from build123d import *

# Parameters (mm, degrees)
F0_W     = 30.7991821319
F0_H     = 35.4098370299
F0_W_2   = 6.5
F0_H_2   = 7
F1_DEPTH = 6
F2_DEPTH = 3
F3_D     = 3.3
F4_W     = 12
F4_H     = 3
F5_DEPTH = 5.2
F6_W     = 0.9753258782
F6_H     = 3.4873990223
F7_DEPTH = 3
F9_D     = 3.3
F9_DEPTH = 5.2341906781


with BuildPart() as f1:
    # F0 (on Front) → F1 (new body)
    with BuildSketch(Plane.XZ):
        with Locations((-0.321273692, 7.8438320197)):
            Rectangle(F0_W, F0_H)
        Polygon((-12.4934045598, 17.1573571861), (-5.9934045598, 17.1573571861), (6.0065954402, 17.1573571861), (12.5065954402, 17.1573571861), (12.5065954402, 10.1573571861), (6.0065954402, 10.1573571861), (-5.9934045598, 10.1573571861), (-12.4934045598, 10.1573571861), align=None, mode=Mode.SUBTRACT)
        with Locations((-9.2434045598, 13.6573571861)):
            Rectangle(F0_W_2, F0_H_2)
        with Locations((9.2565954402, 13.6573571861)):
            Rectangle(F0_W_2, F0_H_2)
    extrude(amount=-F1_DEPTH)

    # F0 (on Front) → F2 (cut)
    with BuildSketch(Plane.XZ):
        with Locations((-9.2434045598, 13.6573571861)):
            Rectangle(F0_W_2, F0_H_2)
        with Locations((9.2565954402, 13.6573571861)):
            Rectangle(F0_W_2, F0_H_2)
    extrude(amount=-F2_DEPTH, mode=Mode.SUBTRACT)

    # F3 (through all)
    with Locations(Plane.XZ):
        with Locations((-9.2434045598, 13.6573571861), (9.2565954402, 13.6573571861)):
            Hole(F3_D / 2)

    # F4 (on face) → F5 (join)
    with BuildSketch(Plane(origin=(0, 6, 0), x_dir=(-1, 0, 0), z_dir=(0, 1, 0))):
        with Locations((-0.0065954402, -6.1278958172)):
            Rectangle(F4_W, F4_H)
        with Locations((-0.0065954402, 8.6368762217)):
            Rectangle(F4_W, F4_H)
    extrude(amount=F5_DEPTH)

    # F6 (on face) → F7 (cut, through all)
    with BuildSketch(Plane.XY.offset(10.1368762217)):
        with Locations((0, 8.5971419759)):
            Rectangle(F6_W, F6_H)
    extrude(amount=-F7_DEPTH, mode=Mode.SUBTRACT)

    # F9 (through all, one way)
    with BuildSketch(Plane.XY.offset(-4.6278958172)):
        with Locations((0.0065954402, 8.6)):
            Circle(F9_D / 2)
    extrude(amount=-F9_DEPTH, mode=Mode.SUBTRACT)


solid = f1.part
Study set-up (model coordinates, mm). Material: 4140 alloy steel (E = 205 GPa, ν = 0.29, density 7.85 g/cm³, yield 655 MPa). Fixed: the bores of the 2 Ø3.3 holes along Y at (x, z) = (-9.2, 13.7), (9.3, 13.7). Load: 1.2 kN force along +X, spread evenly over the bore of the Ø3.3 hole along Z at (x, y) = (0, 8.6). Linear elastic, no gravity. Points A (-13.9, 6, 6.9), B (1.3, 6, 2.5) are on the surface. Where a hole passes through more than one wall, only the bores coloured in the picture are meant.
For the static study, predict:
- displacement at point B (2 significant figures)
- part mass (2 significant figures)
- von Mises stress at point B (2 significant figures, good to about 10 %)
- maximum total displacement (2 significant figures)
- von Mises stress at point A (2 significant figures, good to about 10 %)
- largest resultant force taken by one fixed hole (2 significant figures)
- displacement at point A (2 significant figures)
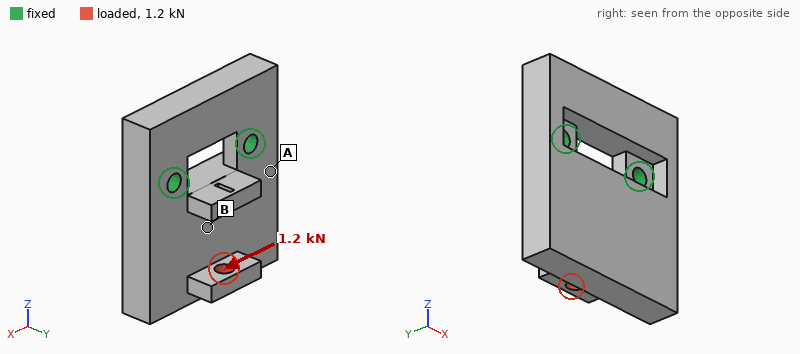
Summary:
4.8 µm
48 g
59 MPa
18 µm
22 MPa
1.2 kN
4.9 µm
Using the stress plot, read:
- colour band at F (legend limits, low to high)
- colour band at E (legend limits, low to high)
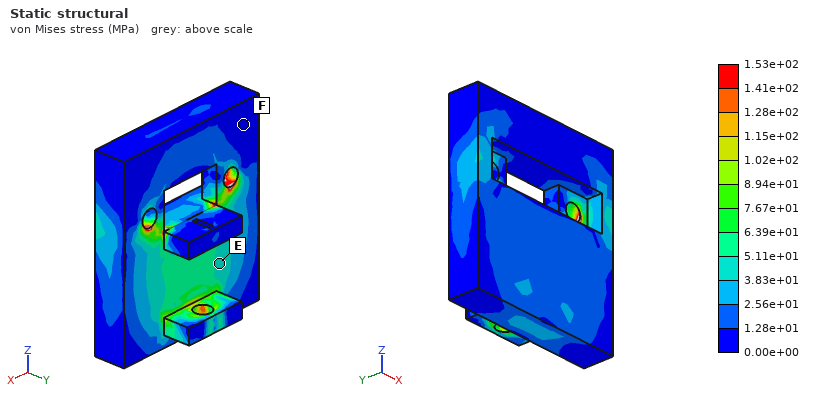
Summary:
0.00e+00 to 1.28e+01 MPa
3.83e+01 to 5.11e+01 MPa
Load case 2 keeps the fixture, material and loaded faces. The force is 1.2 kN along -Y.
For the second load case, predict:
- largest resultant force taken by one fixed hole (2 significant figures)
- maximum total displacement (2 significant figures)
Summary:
620 N
0.14 mm
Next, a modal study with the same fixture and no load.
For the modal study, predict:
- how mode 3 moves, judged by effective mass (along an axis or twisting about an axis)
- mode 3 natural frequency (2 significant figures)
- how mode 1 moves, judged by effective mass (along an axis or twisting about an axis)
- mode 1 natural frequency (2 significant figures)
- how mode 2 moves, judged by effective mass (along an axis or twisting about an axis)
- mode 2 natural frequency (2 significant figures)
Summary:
along Y
14 kHz
along Y
4000 Hz
twisting about Z
12 kHz
